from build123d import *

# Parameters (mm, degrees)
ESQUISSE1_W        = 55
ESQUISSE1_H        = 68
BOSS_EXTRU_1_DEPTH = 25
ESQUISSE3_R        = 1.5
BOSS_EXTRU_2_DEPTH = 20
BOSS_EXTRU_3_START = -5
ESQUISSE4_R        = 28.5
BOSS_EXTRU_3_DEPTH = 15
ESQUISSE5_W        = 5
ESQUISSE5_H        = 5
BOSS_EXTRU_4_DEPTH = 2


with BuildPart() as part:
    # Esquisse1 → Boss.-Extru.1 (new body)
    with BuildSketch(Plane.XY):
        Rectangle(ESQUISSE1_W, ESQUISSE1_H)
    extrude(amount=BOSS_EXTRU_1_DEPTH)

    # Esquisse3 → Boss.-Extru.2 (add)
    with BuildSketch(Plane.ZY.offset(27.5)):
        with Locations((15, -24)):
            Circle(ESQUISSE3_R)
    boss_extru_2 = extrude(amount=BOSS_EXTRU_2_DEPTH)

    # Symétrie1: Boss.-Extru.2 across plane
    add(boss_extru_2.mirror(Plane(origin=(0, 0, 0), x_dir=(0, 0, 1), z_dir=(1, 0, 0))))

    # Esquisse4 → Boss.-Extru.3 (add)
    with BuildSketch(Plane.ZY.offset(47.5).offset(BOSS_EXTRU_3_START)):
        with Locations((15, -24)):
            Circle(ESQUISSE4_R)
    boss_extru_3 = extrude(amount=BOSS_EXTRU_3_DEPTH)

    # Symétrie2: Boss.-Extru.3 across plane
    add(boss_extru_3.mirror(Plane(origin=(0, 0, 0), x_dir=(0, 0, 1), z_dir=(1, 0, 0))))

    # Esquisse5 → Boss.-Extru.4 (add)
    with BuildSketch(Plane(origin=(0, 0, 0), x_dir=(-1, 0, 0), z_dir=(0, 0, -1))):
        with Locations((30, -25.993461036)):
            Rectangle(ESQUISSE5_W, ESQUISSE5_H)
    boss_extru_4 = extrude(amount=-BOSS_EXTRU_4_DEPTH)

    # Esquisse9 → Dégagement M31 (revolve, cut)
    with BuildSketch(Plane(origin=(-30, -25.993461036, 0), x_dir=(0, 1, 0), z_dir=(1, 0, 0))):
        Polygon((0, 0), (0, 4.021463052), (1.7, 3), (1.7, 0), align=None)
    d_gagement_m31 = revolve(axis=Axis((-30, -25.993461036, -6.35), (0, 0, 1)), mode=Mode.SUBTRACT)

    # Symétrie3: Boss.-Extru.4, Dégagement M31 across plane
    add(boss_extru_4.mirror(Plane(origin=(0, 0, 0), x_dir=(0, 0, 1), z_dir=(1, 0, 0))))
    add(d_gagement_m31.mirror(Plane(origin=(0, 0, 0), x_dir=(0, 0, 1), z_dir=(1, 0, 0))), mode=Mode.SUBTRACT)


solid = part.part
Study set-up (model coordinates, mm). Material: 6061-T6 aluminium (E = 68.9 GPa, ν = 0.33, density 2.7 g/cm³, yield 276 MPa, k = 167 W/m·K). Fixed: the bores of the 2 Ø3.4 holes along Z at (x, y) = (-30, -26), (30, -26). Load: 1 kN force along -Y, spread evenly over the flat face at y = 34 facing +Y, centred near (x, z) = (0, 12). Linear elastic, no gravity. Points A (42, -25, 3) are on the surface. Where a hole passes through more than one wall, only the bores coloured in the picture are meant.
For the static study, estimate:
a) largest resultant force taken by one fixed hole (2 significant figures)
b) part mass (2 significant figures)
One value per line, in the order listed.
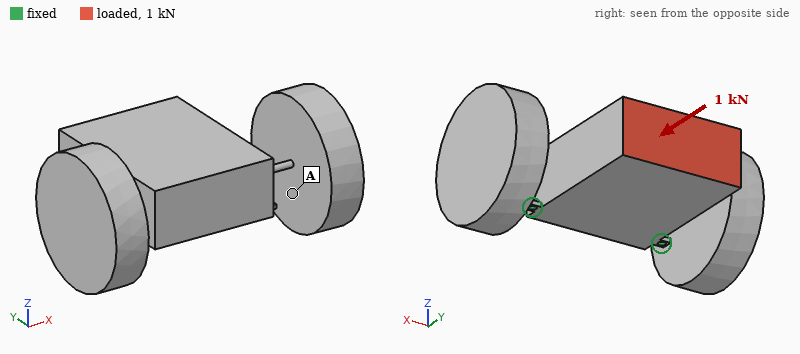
500 N
460 g
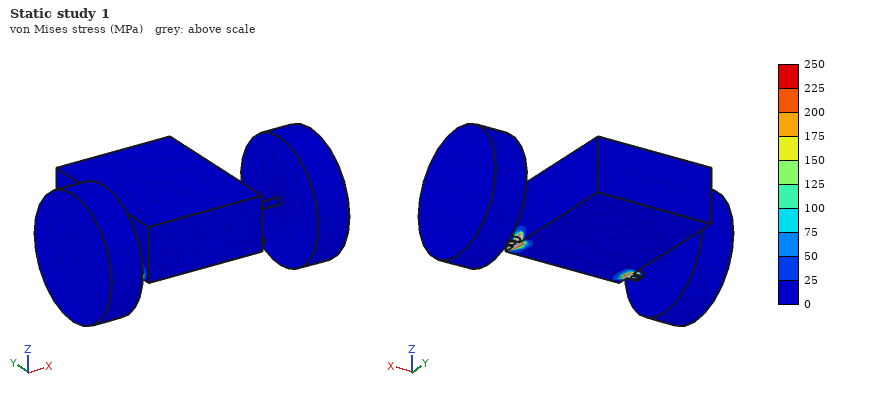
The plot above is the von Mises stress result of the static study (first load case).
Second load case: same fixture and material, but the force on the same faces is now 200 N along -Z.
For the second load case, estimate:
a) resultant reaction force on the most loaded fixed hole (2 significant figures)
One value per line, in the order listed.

110 N
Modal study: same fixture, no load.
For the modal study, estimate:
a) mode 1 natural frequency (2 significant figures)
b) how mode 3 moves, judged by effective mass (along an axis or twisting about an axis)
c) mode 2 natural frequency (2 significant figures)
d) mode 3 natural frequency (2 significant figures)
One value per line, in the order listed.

85 Hz
along Y
89 Hz
94 Hz
